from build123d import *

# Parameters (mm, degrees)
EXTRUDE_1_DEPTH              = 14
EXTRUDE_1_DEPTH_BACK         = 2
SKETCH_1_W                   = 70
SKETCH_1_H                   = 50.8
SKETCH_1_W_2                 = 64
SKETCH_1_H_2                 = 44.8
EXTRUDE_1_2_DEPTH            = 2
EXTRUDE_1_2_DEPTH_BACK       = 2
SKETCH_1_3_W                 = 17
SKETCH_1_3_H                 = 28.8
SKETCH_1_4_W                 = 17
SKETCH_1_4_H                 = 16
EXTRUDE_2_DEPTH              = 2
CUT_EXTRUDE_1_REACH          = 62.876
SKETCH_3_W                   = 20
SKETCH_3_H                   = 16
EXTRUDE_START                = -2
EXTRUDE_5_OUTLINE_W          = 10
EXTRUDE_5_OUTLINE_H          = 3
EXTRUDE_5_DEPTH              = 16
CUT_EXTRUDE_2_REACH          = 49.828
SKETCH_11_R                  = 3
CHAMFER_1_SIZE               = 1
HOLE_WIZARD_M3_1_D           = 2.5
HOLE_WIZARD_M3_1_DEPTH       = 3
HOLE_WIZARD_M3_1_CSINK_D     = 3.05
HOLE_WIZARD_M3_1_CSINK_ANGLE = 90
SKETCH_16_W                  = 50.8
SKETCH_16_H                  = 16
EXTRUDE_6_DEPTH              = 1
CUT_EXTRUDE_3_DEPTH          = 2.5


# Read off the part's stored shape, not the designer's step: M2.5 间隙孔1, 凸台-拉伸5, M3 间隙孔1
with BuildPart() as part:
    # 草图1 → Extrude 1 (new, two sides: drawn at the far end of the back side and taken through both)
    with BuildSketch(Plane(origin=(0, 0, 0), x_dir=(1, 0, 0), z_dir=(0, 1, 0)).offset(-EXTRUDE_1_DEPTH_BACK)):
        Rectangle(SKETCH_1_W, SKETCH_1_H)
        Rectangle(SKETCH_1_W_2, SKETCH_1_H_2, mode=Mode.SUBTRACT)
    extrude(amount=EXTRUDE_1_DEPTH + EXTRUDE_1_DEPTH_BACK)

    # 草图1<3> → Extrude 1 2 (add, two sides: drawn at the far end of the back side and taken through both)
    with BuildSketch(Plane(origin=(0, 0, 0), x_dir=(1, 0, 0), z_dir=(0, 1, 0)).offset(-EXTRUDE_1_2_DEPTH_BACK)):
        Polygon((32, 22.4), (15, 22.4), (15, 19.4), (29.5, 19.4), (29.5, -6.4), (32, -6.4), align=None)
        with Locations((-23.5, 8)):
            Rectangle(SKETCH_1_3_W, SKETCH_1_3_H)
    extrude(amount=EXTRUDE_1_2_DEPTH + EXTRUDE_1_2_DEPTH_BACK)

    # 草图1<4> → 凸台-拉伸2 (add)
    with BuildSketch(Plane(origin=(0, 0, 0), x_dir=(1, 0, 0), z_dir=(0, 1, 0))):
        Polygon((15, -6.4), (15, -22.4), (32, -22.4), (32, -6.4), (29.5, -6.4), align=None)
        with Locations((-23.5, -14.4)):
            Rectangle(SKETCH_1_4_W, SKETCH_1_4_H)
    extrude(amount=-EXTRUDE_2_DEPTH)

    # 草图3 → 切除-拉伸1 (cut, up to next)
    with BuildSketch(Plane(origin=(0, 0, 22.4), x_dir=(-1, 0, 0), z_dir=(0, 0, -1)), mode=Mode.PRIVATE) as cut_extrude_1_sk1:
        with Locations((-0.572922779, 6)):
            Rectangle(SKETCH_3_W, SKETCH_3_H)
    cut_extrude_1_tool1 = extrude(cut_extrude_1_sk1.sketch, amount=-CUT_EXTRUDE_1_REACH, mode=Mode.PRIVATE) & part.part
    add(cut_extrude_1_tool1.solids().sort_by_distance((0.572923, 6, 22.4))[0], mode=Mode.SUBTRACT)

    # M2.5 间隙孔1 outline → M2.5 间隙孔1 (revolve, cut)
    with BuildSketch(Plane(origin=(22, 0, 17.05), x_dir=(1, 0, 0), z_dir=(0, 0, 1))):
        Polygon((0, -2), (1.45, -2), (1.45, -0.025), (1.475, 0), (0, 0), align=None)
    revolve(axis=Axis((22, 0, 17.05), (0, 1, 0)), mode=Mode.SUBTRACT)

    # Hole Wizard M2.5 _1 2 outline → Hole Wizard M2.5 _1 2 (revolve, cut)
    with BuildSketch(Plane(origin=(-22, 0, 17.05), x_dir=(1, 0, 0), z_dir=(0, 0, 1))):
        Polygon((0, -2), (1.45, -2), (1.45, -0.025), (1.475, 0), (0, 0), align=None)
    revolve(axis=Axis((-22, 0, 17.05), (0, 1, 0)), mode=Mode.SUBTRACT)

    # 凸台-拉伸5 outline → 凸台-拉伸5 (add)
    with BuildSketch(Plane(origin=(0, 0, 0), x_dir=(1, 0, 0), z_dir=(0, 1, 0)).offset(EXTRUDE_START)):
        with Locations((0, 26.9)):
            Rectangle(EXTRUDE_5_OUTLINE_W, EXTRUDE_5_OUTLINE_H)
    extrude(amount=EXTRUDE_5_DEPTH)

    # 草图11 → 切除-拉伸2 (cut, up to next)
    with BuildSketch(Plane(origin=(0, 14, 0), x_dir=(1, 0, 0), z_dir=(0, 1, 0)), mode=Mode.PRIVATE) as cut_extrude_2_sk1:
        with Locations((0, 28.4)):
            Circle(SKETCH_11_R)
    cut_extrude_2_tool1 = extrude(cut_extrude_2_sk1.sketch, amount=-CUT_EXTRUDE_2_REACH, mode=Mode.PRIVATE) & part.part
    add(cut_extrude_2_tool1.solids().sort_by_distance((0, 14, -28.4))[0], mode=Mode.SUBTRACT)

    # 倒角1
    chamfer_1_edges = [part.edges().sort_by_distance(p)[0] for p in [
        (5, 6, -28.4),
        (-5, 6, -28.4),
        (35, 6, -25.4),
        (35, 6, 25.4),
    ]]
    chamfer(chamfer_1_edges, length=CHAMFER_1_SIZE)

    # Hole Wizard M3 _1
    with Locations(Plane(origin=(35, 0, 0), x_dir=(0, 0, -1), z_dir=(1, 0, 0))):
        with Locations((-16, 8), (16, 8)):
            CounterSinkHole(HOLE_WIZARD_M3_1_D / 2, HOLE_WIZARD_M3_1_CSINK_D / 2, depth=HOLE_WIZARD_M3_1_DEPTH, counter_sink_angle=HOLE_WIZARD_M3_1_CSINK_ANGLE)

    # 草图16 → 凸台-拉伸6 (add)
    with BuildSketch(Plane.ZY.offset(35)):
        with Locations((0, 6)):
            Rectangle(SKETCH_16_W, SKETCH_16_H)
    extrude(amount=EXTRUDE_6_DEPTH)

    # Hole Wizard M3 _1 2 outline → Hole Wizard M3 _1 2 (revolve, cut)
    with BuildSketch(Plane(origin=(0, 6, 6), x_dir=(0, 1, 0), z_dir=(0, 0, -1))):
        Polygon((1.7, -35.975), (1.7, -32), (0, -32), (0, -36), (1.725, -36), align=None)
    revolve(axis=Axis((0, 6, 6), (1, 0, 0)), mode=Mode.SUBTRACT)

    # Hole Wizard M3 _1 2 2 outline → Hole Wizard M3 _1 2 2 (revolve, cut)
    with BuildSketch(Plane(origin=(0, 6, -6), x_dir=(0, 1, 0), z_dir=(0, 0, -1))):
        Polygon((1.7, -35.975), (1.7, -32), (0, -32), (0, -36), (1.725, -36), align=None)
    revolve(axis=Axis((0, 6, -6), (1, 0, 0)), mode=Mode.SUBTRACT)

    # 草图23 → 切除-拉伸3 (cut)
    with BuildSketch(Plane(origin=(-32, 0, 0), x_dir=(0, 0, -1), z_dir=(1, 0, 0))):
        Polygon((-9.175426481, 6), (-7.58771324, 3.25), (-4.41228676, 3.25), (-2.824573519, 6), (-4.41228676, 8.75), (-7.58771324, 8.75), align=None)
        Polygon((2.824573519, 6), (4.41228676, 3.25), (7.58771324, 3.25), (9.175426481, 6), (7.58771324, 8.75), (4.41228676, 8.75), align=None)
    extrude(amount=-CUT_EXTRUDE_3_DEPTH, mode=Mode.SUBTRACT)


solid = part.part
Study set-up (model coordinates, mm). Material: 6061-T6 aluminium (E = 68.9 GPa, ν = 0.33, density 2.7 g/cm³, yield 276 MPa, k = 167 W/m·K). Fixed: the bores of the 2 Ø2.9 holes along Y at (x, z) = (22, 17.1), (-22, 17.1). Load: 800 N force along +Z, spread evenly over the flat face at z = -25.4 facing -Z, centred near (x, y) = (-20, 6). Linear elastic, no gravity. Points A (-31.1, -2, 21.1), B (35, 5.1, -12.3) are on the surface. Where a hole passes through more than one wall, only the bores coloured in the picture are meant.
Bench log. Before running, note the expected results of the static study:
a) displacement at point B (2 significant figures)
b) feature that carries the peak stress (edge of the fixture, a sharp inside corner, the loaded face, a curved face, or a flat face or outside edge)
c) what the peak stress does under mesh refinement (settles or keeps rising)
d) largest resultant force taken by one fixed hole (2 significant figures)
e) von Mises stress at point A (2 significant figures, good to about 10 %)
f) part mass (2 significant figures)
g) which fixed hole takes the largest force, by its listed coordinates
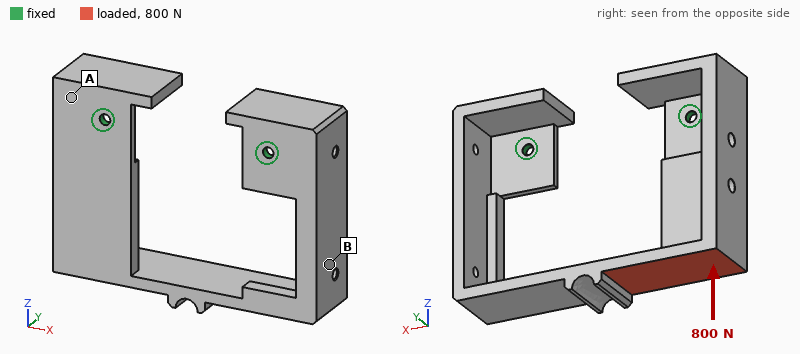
0.22 mm
edge of the fixture
keeps rising
770 N
32 MPa
39 g
(-22, 17.1)
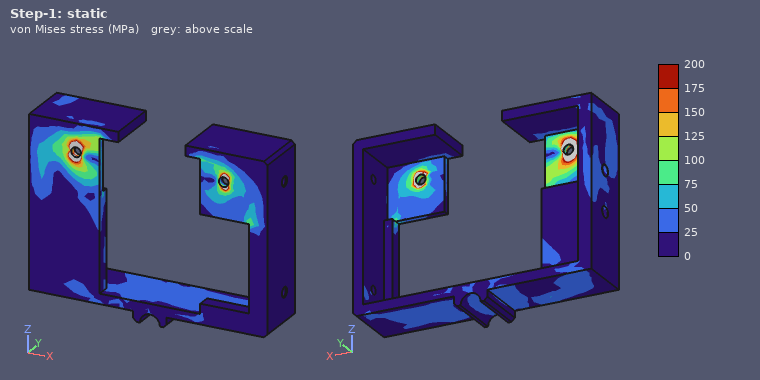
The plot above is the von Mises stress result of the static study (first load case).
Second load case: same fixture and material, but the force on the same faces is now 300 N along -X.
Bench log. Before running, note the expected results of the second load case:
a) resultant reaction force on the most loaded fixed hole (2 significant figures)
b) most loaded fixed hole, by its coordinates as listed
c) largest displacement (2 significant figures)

200 N
(-22, 17.1)
0.27 mm
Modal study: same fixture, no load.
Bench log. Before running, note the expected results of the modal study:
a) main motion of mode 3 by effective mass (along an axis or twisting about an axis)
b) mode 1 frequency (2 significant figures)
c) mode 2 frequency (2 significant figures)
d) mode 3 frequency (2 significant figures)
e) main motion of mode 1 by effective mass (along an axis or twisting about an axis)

along X
670 Hz
1100 Hz
1600 Hz
along Y
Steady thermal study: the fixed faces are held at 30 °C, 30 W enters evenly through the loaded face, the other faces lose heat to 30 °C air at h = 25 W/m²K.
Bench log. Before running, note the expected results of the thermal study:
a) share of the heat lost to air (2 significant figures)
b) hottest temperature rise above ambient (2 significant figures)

23 %
65 K
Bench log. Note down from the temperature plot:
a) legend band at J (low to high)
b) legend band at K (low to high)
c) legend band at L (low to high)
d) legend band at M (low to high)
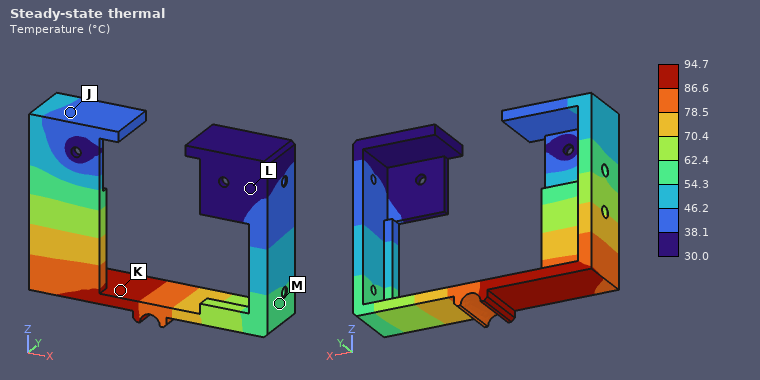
38.1 to 46.2 °C
86.6 to 94.7 °C
30.0 to 38.1 °C
54.3 to 62.4 °C
